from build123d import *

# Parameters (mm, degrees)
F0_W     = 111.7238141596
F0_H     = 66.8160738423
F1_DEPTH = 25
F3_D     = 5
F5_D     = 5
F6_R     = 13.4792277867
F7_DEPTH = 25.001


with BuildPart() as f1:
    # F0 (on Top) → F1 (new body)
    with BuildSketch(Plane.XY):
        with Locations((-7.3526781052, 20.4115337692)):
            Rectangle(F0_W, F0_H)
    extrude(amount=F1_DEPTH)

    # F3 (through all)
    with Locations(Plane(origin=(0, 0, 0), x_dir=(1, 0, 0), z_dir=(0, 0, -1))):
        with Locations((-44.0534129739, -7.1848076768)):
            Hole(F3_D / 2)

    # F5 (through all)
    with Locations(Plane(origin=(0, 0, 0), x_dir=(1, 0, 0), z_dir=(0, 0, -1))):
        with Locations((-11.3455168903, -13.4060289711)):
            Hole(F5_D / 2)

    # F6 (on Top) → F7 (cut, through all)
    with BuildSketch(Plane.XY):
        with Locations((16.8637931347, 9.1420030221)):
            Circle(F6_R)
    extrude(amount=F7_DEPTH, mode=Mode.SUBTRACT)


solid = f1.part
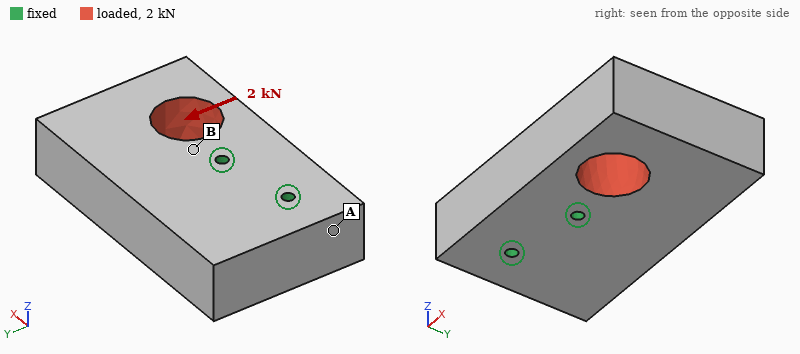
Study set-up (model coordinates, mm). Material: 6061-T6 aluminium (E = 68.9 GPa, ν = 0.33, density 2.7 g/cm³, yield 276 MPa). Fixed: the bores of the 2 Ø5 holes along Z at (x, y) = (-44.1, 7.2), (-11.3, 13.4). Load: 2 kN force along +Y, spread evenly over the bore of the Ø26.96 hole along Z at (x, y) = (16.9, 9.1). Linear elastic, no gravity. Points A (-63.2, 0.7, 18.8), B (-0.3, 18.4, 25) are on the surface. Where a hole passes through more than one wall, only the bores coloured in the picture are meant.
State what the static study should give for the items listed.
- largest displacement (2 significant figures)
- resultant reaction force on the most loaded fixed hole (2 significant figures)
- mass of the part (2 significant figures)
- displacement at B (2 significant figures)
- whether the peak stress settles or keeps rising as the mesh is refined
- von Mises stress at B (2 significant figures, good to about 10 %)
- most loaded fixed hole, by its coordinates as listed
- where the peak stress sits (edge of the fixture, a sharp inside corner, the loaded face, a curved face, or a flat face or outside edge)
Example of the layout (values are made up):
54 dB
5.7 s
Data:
11 µm
3.5 kN
460 g
2.1 µm
keeps rising
3.5 MPa
(-11.3, 13.4)
edge of the fixture
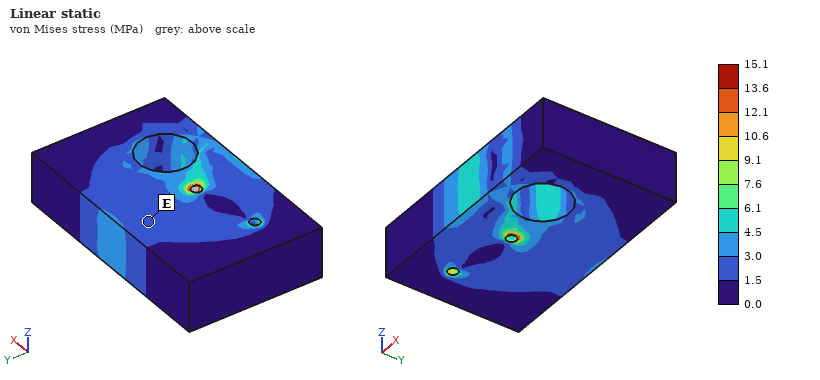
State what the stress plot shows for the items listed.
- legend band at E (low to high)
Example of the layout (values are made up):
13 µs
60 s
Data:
1.5 to 3.0 MPa
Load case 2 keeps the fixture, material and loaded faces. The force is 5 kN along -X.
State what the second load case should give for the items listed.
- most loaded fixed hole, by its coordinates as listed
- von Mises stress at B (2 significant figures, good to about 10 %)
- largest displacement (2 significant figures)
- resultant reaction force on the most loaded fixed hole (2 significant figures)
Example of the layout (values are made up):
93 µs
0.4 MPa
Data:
(-11.3, 13.4)
7.8 MPa
6.6 µm
3.3 kN
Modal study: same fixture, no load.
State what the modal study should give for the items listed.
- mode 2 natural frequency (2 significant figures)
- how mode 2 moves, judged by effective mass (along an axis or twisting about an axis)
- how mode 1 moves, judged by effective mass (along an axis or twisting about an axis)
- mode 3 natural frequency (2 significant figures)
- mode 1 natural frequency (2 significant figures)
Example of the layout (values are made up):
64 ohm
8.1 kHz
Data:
4700 Hz
along Y
along Z
5500 Hz
3500 Hz
